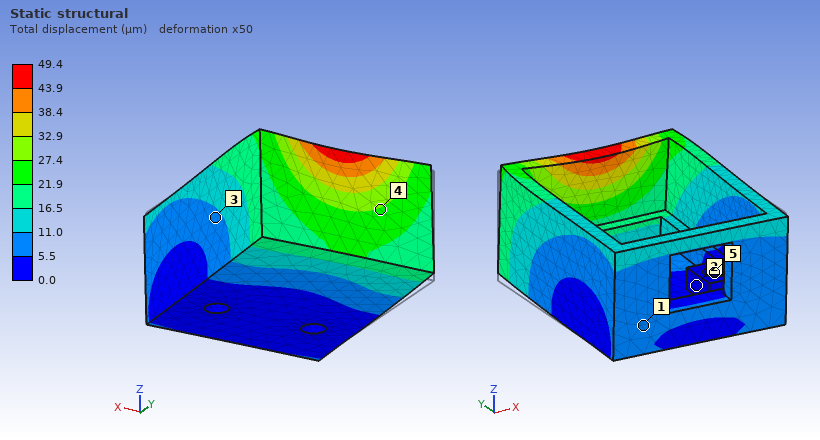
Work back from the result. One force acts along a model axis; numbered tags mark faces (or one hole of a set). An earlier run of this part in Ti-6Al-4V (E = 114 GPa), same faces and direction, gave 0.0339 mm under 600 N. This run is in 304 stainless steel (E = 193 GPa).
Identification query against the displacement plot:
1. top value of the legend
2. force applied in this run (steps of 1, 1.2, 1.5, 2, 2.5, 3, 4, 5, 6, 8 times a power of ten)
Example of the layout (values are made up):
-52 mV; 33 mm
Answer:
49.4 µm; 1.5 kN
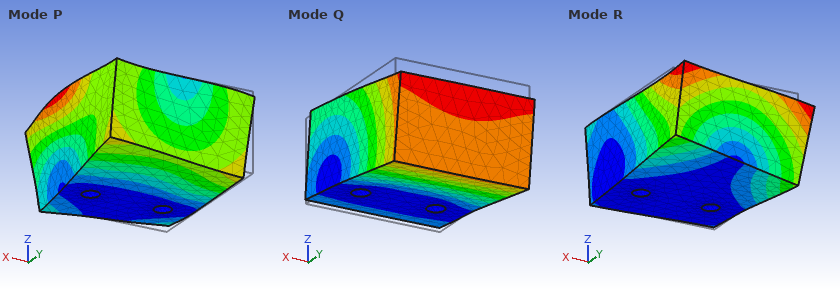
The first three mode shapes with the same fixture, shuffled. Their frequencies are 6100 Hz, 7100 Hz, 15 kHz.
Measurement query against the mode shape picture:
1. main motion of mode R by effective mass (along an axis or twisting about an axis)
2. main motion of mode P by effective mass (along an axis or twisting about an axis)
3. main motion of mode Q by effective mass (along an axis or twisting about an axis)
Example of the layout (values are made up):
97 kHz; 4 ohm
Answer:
along X; along X; along Z
